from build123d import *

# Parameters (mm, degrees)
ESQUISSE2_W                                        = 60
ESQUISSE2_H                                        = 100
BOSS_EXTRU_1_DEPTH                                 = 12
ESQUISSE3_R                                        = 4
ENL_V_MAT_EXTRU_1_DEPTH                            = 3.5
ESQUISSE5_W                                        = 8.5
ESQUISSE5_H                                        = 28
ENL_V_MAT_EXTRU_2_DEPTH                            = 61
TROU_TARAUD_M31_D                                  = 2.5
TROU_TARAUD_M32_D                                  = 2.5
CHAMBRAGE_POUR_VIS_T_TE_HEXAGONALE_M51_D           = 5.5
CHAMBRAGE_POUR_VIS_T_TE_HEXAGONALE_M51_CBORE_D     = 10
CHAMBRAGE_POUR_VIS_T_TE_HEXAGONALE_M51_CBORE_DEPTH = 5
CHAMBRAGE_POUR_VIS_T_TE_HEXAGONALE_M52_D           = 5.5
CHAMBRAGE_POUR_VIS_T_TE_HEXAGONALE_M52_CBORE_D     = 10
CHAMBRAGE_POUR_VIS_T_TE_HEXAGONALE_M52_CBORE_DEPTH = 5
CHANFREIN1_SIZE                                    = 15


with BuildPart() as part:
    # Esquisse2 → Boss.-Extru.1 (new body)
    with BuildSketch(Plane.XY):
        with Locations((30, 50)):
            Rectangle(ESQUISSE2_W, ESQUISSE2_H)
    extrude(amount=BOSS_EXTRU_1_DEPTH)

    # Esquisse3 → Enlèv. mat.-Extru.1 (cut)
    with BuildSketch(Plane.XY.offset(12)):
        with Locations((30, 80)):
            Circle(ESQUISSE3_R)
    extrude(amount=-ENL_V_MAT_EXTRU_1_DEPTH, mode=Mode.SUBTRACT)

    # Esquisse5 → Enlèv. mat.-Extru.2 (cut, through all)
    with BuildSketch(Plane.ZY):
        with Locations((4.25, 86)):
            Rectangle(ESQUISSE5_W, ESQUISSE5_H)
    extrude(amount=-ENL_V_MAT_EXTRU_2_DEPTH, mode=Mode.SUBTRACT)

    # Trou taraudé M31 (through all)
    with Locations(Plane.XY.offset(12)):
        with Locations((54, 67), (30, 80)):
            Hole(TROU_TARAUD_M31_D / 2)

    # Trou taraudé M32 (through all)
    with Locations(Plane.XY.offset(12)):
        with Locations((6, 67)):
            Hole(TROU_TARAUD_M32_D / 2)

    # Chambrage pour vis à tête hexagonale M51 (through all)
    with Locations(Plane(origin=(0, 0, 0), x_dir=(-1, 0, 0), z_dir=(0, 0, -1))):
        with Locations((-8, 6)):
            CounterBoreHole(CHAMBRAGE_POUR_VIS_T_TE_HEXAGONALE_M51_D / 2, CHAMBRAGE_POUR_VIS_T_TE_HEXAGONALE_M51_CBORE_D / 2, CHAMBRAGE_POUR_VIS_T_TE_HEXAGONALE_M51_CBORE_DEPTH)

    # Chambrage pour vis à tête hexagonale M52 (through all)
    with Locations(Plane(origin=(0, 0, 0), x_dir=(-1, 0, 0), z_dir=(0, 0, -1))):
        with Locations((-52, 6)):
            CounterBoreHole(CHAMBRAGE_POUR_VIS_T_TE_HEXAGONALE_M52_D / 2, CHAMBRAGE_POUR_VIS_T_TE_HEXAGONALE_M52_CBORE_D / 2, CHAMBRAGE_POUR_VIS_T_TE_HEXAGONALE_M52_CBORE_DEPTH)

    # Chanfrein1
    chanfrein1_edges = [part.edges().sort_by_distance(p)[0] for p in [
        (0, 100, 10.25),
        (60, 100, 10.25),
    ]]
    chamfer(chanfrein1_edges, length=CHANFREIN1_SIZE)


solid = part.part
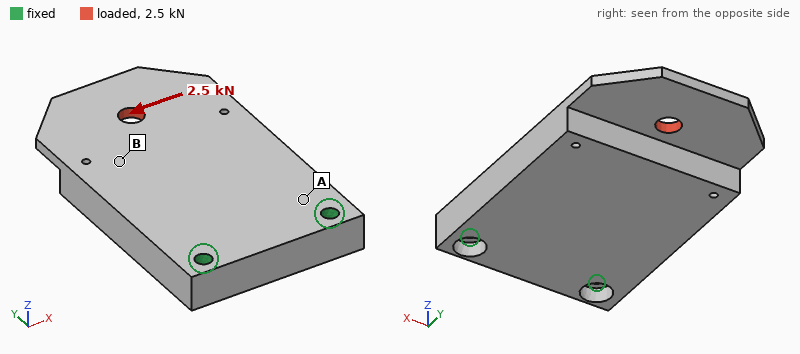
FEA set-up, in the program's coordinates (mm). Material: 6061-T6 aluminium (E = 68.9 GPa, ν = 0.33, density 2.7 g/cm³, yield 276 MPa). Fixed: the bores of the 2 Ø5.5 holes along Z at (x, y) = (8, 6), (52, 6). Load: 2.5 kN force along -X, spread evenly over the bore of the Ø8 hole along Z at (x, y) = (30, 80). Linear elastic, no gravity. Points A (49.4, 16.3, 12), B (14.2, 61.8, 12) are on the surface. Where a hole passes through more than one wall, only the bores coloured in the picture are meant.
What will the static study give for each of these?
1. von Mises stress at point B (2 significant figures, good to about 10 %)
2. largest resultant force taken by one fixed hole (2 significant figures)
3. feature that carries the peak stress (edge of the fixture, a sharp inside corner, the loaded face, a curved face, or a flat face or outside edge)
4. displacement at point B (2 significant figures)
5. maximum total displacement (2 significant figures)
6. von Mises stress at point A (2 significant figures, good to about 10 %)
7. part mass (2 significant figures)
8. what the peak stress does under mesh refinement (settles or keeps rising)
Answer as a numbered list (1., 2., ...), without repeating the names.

1. 12 MPa
2. 4.2 kN
3. edge of the fixture
4. 39 µm
5. 69 µm
6. 29 MPa
7. 150 g
8. keeps rising
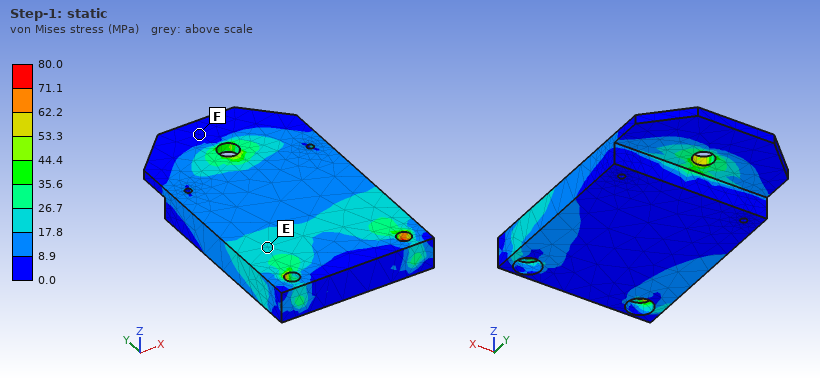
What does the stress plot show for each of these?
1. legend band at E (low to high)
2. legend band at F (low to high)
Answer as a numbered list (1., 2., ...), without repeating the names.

1. 17.8 to 26.7 MPa
2. 0.0 to 8.9 MPa
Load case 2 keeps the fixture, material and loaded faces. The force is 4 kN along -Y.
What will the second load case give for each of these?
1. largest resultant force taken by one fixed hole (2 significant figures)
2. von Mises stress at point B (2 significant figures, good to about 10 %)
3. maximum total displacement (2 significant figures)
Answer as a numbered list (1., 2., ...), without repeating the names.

1. 2.0 kN
2. 19 MPa
3. 0.15 mm
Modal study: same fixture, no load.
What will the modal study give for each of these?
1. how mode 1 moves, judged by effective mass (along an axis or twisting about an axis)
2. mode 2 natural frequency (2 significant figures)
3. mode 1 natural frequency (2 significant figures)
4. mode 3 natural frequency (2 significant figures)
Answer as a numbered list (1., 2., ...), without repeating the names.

1. along Z
2. 4000 Hz
3. 1100 Hz
4. 4100 Hz
